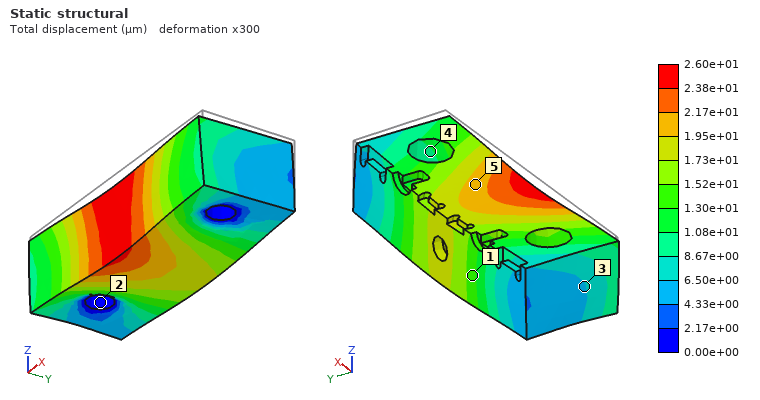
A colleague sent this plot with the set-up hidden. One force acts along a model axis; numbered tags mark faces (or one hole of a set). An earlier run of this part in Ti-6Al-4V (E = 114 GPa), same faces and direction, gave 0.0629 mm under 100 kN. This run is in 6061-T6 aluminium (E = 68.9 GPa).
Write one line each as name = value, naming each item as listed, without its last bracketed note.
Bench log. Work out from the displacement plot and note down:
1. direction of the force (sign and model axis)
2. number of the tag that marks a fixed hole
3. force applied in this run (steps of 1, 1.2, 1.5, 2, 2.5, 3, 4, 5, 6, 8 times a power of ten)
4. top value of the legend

direction of the force = -Z
number of the tag that marks a fixed hole = 2
force applied in this run = 25 kN
top value of the legend = 2.60e+01 µm
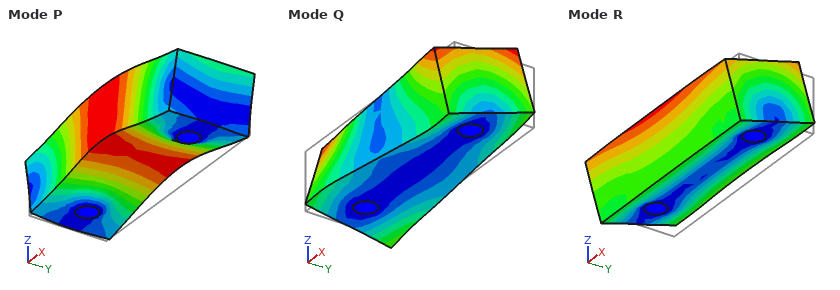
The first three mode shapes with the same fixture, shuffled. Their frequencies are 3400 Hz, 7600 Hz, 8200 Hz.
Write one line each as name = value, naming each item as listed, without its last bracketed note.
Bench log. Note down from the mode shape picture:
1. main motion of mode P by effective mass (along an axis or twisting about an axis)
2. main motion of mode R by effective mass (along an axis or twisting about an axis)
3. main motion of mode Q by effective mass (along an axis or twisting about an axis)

main motion of mode P by effective mass = along Z
main motion of mode R by effective mass = along Y
main motion of mode Q by effective mass = twisting about Z
